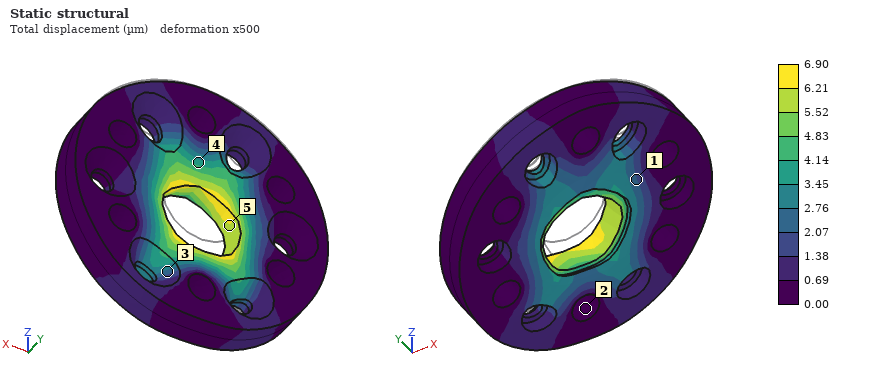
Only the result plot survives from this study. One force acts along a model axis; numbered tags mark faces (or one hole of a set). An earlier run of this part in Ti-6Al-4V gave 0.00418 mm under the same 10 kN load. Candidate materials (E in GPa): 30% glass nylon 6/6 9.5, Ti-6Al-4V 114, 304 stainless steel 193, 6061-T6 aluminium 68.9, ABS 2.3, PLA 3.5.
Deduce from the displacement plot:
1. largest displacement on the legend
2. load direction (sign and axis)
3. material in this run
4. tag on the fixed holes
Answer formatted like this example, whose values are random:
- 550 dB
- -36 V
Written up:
- 6.90 µm
- -Z
- 6061-T6 aluminium
- 2
